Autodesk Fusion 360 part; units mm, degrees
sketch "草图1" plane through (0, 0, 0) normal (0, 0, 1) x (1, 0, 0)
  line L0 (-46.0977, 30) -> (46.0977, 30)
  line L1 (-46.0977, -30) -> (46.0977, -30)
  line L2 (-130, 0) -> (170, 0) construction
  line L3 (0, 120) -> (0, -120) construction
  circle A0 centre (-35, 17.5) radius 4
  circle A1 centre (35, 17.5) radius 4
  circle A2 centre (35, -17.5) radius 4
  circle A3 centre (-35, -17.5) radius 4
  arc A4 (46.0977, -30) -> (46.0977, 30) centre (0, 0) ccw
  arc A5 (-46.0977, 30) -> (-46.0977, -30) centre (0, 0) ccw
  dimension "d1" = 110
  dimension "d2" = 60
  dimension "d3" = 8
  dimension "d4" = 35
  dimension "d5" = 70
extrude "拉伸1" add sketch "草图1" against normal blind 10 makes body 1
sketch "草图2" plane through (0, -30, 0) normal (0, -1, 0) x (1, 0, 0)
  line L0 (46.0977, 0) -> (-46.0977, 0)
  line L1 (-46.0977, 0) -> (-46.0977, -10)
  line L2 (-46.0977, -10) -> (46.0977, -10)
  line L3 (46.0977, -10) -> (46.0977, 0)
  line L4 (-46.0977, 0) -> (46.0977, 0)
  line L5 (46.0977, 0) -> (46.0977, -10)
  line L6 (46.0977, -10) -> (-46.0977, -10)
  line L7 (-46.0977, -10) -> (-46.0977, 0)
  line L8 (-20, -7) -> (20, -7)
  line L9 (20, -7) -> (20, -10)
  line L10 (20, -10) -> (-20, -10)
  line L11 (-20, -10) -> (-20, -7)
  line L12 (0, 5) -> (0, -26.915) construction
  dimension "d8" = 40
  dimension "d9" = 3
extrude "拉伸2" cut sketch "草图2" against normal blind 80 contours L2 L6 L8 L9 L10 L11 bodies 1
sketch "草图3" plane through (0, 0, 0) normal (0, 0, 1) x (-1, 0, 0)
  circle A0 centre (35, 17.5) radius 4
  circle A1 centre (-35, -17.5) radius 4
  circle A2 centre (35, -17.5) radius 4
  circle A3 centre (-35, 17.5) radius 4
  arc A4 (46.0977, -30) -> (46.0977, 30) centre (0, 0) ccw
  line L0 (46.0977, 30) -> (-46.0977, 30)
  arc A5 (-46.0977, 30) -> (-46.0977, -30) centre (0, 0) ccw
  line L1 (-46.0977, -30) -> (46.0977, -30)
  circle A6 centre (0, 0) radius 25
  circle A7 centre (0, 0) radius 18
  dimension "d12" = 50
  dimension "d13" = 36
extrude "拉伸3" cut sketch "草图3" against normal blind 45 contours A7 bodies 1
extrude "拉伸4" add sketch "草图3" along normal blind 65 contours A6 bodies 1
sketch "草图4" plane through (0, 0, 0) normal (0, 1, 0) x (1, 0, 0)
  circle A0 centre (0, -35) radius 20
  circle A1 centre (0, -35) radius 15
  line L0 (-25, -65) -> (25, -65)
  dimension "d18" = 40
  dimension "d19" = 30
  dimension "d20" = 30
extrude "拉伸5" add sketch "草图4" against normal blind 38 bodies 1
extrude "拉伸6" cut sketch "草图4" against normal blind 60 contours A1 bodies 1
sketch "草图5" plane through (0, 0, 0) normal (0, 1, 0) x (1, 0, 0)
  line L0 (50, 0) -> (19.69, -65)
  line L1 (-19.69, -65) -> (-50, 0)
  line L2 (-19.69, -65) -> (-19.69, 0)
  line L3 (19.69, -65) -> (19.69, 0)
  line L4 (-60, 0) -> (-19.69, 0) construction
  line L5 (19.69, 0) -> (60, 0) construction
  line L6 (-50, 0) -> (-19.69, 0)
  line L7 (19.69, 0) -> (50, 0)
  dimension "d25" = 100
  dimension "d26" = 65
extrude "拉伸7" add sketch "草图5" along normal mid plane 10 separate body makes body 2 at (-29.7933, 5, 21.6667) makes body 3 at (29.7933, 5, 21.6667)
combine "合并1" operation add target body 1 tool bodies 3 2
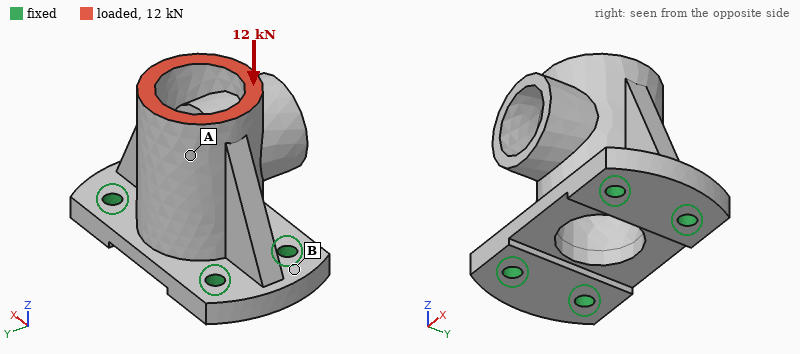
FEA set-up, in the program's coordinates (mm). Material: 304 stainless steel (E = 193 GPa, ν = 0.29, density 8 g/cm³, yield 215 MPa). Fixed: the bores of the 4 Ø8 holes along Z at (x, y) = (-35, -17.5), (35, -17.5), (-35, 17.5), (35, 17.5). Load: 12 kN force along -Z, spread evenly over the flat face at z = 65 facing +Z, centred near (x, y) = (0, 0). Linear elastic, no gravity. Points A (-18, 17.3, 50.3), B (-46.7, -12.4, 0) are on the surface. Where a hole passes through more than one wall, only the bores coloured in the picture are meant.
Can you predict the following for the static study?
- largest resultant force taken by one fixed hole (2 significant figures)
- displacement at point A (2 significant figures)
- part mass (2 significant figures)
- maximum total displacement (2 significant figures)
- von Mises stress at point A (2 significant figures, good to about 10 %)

3.3 kN
7.1 µm
1.1 kg
14 µm
13 MPa
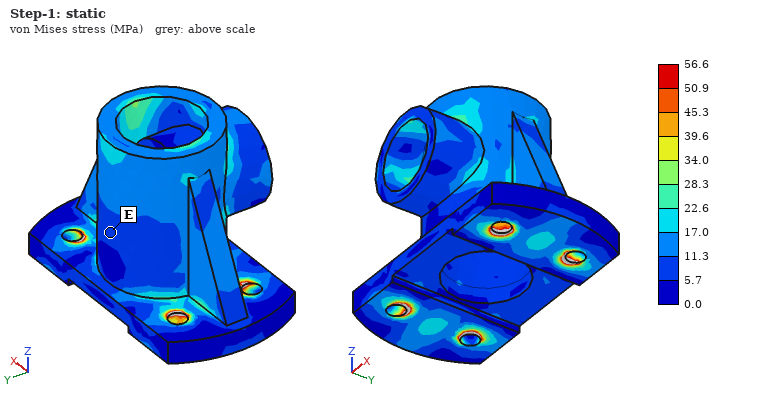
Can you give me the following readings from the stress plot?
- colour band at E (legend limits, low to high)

5.7 to 11.3 MPa
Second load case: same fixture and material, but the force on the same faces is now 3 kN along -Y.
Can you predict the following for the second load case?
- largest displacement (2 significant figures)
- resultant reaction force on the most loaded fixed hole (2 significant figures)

50 µm
3.4 kN
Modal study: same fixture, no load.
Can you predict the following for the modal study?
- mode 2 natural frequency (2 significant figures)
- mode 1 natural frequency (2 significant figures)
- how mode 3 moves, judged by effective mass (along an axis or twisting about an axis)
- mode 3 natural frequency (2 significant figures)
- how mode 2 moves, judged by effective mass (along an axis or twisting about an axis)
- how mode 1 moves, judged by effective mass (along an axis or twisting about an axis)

5600 Hz
2700 Hz
along Z
7900 Hz
along X
along Y
